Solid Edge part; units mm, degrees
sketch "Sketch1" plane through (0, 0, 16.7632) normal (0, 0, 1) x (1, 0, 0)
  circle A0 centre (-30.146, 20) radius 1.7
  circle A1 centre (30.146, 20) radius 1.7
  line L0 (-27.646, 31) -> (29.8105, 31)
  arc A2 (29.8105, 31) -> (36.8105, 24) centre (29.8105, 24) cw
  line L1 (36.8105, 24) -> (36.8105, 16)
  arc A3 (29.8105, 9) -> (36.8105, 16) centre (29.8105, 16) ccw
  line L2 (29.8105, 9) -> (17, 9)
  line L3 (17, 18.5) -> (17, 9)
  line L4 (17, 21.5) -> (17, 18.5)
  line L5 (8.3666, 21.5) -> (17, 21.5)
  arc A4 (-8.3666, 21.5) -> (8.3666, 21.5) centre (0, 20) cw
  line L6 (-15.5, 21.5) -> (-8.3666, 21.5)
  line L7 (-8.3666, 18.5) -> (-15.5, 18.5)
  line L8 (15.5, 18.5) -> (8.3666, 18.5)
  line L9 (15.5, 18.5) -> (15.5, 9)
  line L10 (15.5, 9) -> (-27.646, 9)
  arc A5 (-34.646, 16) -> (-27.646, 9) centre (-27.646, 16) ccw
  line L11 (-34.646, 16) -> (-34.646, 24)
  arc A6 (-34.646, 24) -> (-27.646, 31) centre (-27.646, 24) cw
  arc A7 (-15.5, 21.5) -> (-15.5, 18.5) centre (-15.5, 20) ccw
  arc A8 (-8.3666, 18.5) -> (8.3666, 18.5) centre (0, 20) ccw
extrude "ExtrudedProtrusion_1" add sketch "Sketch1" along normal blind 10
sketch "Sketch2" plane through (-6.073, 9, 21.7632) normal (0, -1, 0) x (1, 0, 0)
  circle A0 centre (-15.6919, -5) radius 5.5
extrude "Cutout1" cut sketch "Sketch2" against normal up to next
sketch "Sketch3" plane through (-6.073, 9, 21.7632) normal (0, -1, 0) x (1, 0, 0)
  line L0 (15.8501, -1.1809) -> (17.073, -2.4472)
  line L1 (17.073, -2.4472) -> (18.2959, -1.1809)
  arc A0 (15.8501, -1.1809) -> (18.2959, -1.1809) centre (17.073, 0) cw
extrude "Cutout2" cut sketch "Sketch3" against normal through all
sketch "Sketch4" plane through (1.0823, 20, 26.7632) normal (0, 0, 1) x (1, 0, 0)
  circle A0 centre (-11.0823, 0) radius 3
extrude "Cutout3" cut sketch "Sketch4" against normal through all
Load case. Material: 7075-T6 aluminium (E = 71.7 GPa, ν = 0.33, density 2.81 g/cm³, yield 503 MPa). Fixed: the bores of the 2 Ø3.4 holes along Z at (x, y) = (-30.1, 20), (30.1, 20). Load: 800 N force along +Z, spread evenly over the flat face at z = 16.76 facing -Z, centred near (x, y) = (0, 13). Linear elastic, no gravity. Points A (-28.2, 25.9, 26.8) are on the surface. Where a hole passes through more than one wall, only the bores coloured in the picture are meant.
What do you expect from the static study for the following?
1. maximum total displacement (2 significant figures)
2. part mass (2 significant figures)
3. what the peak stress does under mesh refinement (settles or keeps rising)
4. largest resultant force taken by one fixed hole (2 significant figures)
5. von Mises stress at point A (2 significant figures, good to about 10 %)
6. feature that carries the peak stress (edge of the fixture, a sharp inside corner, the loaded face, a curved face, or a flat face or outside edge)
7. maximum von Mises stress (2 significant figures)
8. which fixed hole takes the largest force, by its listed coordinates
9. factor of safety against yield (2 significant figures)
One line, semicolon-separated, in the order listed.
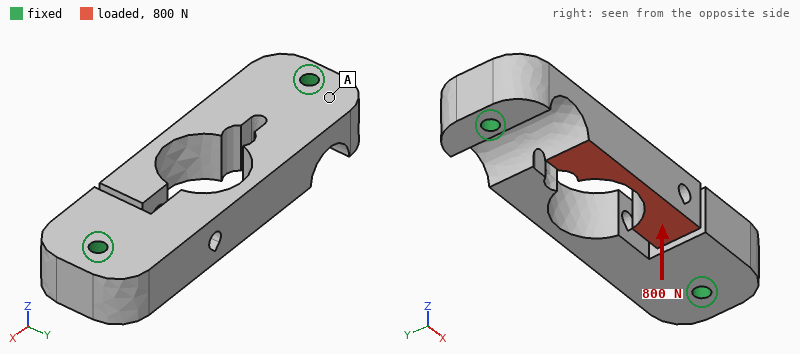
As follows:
0.85 mm; 31 g; settles; 660 N; 43 MPa; a curved face; 560 MPa; (-30.1, 20); 0.91
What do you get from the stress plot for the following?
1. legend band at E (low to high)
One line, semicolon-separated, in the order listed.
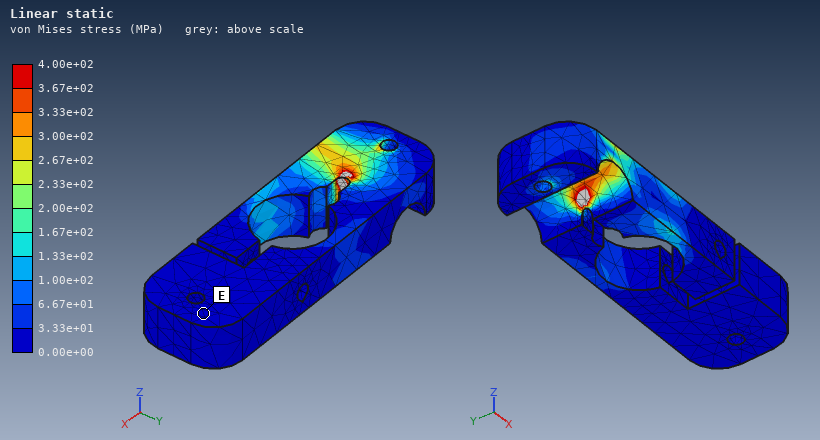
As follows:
0.00e+00 to 3.33e+01 MPa
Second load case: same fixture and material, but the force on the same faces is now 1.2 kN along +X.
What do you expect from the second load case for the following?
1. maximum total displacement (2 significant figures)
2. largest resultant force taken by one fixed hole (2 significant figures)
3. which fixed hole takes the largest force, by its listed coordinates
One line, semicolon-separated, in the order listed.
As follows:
0.47 mm; 1.3 kN; (-30.1, 20)
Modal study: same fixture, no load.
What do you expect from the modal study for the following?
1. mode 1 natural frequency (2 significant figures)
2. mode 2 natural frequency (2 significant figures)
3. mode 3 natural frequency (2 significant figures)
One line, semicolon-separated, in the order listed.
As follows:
2500 Hz; 2600 Hz; 8500 Hz
